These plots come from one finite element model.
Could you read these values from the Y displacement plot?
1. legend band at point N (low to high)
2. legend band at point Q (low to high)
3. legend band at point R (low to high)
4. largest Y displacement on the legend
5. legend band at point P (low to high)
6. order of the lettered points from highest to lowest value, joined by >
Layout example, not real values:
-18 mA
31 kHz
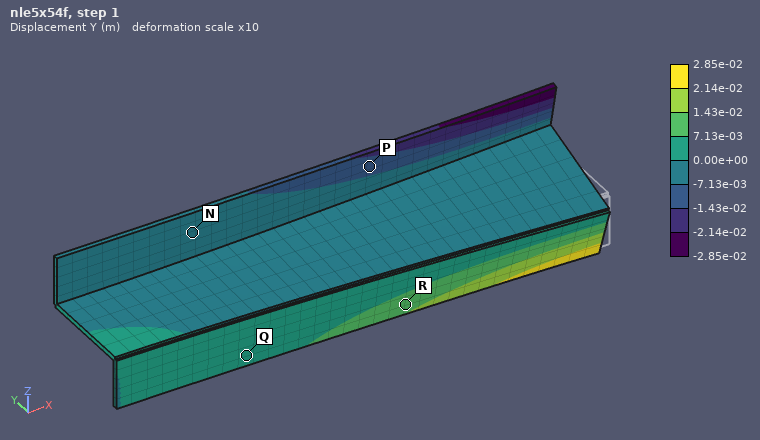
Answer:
-7.13e-03 to 0.00e+00 m
0.00e+00 to 7.13e-03 m
7.13e-03 to 1.43e-02 m
2.85e-02 m
-1.43e-02 to -7.13e-03 m
R > Q > N > P
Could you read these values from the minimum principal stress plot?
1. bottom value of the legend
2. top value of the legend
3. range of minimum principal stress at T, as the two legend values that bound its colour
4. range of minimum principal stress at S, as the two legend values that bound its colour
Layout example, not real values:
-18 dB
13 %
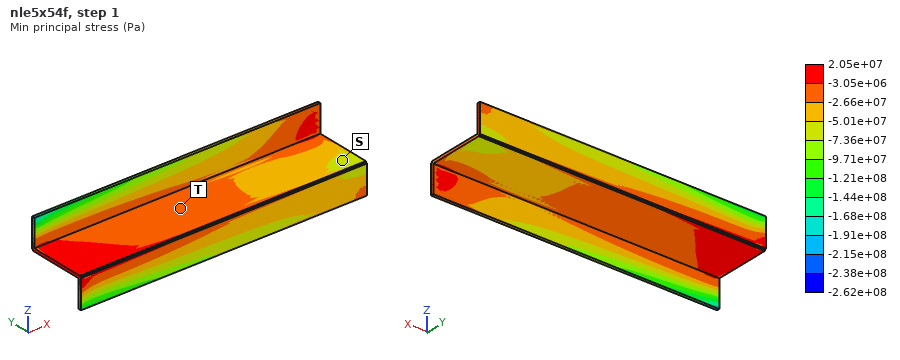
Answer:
-2.62e+08 Pa
2.05e+07 Pa
-2.66e+07 to -3.05e+06 Pa
-7.36e+07 to -5.01e+07 Pa
